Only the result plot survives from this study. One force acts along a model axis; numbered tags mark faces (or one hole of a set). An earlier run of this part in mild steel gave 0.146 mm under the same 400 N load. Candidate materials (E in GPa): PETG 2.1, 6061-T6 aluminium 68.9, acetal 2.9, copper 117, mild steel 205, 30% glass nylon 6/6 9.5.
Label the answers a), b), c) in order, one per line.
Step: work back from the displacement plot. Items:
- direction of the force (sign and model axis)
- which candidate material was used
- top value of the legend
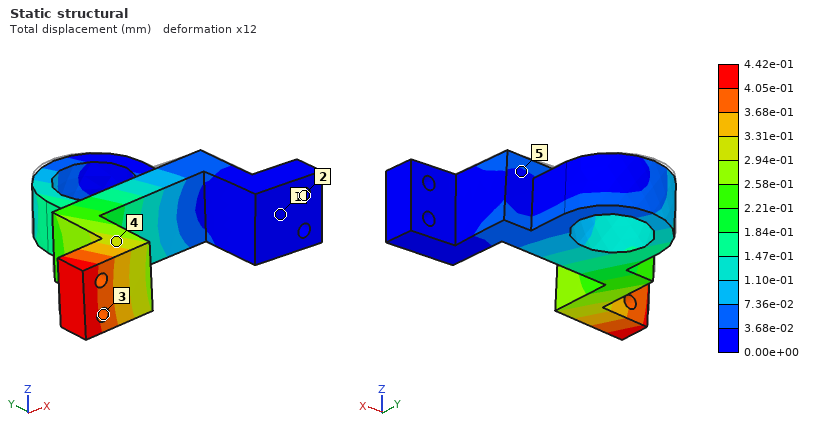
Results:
a) -Z
b) 6061-T6 aluminium
c) 4.42e-01 mm
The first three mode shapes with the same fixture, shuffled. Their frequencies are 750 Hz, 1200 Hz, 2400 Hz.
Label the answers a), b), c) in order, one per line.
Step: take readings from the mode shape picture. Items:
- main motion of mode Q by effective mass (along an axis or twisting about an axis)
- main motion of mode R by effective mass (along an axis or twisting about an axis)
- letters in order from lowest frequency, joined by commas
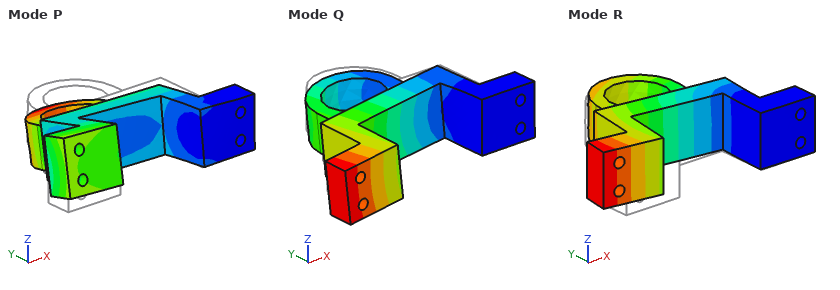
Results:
a) along Z
b) along Y
c) R, Q, P
